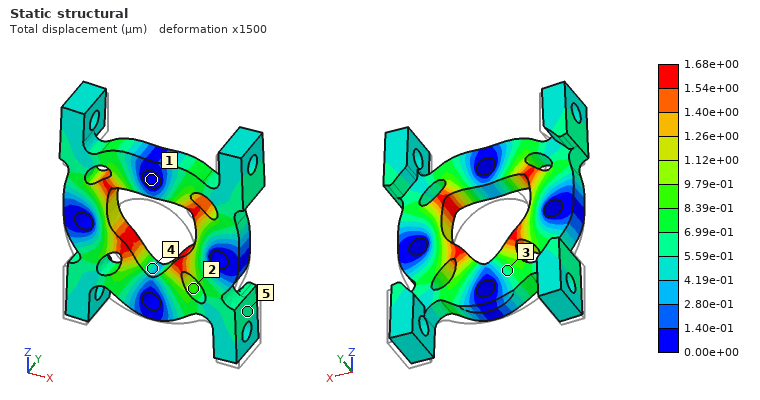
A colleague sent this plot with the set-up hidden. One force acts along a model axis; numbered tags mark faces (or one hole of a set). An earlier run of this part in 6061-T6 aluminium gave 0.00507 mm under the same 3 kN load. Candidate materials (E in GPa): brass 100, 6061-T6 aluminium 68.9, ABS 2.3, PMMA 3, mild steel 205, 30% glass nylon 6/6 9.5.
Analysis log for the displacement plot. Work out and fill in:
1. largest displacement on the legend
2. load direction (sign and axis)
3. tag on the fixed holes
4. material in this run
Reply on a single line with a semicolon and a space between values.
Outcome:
1.68e+00 µm; +Z; 1; mild steel
